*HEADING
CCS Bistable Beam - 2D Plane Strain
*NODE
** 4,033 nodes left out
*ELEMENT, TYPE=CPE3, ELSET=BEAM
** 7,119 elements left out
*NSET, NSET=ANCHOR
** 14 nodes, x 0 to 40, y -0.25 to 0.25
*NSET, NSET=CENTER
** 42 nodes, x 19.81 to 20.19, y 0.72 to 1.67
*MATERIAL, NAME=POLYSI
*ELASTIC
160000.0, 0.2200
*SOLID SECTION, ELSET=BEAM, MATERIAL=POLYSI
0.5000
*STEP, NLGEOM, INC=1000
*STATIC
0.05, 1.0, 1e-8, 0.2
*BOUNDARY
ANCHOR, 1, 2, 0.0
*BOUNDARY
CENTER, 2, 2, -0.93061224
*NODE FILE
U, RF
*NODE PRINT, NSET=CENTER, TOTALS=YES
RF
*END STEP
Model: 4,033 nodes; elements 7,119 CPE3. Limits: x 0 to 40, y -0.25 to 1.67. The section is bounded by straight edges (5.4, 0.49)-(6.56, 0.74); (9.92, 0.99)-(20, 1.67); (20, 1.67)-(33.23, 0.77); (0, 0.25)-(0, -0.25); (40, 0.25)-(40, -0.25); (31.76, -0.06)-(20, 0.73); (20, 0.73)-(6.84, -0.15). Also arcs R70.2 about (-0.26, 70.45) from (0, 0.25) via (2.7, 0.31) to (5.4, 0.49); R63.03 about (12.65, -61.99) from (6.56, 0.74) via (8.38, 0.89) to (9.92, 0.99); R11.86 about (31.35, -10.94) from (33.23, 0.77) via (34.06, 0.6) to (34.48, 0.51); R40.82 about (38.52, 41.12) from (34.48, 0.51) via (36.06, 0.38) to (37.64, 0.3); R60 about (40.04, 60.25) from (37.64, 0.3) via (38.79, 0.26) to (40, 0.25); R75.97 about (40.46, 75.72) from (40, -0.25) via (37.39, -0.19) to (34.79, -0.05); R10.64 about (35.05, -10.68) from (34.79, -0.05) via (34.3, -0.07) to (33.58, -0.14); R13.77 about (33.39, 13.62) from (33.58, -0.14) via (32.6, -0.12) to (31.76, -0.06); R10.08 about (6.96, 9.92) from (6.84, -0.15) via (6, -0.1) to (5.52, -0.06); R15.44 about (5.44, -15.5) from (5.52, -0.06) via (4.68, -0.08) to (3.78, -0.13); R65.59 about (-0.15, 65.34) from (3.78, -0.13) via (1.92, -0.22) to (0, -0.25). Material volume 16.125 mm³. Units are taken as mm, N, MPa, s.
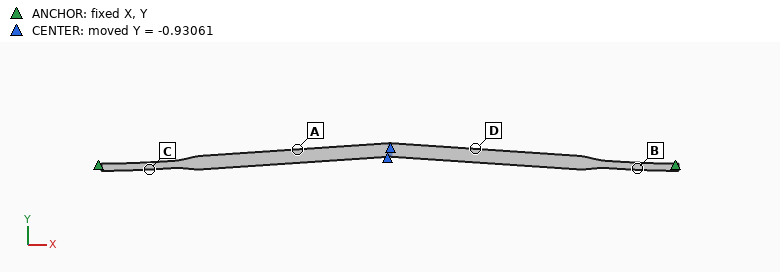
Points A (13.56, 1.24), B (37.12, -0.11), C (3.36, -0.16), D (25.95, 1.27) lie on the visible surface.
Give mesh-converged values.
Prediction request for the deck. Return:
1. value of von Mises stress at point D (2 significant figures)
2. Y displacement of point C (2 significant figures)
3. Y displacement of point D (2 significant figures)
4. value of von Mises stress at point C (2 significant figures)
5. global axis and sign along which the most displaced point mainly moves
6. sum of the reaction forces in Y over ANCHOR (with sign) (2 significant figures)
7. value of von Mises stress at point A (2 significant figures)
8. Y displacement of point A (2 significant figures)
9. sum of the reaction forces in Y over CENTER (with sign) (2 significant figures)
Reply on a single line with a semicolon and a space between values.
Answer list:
630 MPa; -0.14 mm; -0.81 mm; 690 MPa; -Y; 8.8 N; 620 MPa; -0.79 mm; -8.8 N
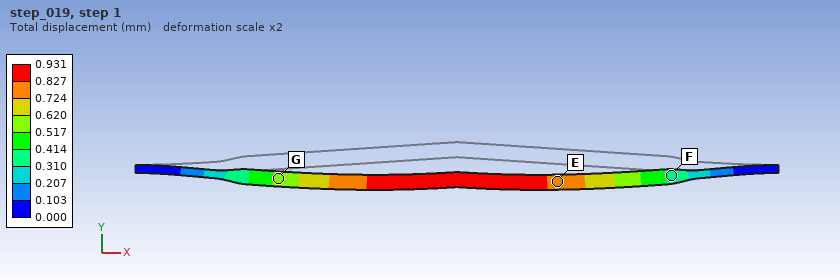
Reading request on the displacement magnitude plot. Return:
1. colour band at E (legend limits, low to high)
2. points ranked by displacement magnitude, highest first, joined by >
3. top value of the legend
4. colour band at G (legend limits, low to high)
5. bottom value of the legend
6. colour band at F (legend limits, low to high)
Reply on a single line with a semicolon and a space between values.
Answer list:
0.724 to 0.827 mm; E > G > F; 0.931 mm; 0.517 to 0.620 mm; 0.000 mm; 0.310 to 0.414 mm
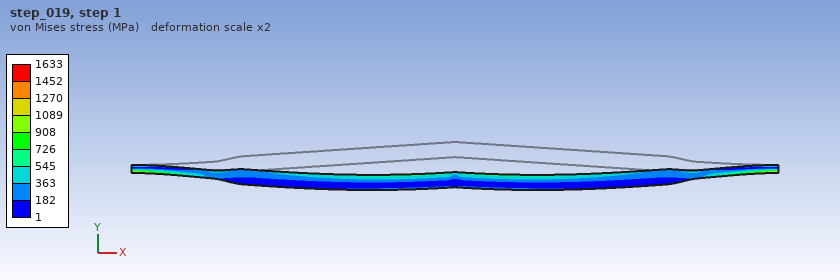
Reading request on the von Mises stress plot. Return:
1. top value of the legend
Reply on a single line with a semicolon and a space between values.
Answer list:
1633 MPa
